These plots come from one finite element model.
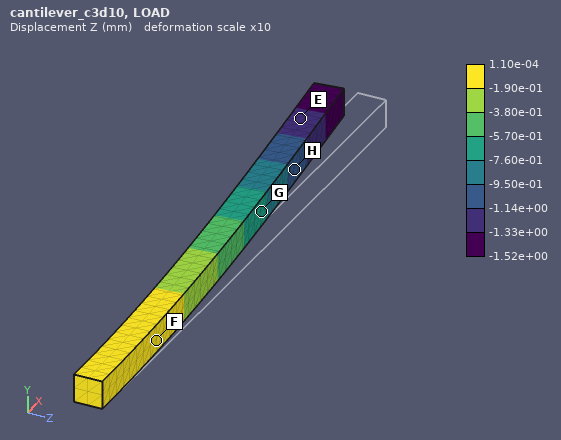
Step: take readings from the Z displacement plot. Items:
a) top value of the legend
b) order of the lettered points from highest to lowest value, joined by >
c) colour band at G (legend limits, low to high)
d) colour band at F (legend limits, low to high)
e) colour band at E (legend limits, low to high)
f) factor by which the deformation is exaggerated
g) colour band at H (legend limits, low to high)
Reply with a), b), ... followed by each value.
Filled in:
a) 1.10e-04 mm
b) F > G > H > E
c) -7.60e-01 to -5.70e-01 mm
d) -1.90e-01 to 1.10e-04 mm
e) -1.33e+00 to -1.14e+00 mm
f) 10
g) -1.14e+00 to -9.50e-01 mm
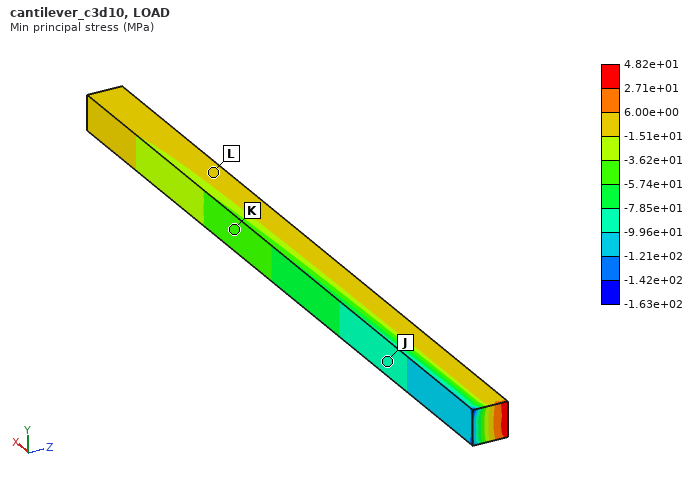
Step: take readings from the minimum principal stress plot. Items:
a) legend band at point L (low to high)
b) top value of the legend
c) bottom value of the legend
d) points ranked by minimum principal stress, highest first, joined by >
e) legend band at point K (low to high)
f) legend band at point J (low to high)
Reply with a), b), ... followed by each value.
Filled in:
a) -1.51e+01 to 6.00e+00 MPa
b) 4.82e+01 MPa
c) -1.63e+02 MPa
d) L > K > J
e) -5.74e+01 to -3.62e+01 MPa
f) -9.96e+01 to -7.85e+01 MPa
